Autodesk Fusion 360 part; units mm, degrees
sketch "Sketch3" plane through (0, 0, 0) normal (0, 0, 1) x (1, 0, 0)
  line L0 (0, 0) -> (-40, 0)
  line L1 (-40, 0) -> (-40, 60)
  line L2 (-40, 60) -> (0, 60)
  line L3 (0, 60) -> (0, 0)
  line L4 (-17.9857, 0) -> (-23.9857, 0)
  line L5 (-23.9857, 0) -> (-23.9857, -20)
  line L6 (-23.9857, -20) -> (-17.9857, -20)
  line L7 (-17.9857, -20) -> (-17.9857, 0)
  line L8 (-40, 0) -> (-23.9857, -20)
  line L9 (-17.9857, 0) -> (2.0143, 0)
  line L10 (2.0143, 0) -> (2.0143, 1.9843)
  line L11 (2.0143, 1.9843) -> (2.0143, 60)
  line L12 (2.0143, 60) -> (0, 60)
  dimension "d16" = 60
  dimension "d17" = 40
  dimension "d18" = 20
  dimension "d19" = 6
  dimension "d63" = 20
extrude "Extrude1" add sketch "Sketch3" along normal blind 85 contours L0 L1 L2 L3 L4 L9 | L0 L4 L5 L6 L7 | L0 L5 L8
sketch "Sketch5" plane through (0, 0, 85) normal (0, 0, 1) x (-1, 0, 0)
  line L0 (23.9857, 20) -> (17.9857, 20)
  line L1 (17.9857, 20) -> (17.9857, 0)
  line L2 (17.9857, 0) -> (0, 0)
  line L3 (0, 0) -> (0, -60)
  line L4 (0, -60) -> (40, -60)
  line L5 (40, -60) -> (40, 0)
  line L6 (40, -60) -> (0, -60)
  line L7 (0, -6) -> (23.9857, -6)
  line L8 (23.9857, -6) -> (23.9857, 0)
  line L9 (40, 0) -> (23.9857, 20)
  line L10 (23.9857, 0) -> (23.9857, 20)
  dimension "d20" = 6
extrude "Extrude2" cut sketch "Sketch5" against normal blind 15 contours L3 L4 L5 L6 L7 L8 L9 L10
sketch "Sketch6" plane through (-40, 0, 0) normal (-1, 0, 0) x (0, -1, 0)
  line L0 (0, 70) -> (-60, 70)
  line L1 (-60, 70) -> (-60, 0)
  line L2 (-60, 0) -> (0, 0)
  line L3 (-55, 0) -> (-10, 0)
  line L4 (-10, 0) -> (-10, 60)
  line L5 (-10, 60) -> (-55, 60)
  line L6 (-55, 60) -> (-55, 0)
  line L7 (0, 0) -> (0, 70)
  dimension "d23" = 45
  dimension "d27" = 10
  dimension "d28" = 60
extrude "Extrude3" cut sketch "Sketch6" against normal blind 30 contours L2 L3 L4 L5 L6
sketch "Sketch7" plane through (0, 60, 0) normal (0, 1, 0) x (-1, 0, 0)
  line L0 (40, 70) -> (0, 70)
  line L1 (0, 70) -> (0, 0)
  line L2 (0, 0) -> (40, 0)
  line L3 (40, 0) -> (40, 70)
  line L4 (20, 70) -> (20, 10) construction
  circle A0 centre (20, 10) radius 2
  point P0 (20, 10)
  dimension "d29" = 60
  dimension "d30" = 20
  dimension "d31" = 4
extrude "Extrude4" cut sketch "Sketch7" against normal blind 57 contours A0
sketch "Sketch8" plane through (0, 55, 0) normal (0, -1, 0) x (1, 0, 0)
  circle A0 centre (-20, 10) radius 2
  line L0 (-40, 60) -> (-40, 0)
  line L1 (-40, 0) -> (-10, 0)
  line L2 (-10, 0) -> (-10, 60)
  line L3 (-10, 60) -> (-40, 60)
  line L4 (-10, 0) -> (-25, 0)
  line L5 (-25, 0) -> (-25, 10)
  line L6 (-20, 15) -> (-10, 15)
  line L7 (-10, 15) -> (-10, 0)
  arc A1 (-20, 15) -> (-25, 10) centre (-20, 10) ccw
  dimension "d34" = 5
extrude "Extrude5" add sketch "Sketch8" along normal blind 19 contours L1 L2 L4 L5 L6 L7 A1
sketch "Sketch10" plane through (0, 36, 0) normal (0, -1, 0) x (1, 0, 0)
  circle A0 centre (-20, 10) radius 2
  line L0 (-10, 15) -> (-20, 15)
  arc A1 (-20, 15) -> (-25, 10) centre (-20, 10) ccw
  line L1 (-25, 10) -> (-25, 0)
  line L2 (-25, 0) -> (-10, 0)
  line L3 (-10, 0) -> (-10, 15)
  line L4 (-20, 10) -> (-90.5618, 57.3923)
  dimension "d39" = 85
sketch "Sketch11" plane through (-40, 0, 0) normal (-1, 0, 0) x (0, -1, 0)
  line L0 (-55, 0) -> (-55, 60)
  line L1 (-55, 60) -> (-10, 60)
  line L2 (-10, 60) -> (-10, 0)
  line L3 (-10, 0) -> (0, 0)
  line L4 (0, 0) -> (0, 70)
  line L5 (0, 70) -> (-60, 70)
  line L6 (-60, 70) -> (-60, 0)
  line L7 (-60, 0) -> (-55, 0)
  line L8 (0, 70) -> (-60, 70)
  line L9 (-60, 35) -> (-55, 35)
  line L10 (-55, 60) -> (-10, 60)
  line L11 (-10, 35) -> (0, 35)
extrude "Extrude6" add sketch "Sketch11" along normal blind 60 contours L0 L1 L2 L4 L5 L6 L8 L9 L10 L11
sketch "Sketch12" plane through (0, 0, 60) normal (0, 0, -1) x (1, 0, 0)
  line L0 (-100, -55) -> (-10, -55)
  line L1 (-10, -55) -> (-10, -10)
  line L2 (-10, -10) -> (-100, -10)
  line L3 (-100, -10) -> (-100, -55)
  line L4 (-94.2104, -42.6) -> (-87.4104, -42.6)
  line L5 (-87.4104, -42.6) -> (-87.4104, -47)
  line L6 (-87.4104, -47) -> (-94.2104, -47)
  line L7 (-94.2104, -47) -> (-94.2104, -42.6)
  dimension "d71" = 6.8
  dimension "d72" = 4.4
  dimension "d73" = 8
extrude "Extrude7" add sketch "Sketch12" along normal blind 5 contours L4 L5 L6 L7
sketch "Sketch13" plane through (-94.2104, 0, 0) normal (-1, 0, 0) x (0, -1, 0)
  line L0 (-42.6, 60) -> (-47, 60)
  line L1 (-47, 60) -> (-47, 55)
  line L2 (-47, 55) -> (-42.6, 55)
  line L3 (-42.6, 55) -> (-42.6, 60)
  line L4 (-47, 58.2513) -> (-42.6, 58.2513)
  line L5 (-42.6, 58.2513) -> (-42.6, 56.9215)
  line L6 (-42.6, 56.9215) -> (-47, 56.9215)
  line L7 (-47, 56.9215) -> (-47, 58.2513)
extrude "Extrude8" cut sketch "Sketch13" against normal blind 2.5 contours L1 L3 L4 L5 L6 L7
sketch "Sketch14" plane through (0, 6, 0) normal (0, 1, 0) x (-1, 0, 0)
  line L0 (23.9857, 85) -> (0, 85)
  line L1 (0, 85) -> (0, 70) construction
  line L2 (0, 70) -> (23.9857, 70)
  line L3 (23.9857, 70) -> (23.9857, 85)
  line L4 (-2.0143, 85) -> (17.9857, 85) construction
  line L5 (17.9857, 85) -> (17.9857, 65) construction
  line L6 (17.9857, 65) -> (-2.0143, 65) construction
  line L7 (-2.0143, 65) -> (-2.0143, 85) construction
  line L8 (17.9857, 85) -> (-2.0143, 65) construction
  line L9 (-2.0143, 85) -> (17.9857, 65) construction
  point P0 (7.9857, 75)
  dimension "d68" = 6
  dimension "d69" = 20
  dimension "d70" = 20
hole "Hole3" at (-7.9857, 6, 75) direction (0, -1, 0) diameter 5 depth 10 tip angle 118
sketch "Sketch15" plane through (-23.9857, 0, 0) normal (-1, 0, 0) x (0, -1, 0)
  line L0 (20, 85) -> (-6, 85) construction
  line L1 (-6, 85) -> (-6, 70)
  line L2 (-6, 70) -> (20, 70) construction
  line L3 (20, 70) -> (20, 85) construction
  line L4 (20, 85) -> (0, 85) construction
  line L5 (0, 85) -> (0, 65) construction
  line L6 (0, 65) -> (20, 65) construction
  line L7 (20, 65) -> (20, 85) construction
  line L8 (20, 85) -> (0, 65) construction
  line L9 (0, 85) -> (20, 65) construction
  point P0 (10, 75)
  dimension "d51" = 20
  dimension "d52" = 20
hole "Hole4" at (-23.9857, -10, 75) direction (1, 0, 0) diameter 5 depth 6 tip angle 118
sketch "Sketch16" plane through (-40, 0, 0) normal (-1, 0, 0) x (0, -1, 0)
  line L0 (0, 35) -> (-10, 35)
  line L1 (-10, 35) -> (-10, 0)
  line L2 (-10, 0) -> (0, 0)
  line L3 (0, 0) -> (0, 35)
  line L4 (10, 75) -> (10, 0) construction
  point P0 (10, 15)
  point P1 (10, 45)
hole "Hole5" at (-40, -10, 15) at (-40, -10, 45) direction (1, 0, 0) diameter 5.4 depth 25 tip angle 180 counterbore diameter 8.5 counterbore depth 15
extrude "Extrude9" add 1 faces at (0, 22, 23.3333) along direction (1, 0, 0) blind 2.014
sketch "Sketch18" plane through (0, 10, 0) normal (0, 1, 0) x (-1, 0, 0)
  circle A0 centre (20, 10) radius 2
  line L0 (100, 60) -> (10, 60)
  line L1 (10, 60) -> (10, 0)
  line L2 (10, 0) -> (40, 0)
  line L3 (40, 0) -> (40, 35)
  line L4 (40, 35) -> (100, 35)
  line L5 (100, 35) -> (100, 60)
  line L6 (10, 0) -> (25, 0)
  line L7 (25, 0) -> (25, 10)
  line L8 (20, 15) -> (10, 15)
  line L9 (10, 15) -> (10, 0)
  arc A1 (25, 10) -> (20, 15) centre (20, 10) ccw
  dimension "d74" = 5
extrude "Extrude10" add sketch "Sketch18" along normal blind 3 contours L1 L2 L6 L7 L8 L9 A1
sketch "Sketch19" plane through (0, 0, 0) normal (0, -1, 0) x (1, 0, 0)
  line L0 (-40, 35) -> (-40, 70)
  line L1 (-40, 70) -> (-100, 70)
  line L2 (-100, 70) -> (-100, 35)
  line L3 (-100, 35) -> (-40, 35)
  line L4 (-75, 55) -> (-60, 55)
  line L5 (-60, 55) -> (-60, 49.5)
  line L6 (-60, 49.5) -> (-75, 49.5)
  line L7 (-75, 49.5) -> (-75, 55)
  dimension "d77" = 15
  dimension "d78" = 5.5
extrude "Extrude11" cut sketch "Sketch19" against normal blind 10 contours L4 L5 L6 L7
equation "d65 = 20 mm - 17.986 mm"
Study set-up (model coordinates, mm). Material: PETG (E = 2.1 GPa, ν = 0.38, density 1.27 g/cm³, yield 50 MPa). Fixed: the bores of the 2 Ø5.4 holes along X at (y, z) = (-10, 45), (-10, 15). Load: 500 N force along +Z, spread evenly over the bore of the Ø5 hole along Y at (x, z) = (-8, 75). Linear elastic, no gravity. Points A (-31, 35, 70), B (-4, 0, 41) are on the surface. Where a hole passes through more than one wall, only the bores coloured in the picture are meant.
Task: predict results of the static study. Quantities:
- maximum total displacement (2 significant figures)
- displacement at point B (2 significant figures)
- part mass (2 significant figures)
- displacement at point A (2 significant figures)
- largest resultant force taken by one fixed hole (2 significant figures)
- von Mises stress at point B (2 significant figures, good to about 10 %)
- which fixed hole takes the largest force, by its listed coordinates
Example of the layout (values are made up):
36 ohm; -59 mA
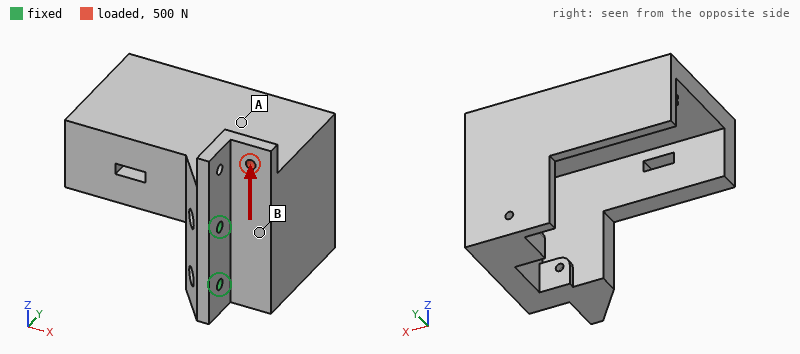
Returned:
0.22 mm; 0.076 mm; 230 g; 0.12 mm; 410 N; 1.3 MPa; (-10, 45)
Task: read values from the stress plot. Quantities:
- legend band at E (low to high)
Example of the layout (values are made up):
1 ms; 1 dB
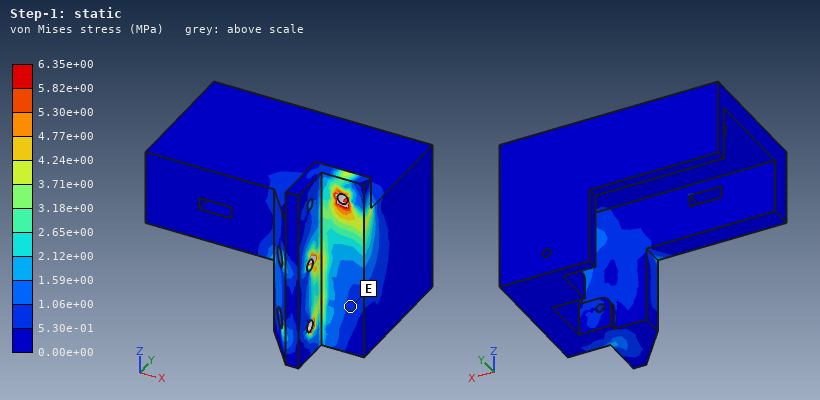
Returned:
5.30e-01 to 1.06e+00 MPa
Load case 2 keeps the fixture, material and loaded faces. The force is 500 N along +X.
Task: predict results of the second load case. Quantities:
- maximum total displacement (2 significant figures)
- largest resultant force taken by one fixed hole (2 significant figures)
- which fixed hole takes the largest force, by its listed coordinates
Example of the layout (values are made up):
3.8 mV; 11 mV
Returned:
1.2 mm; 900 N; (-10, 45)
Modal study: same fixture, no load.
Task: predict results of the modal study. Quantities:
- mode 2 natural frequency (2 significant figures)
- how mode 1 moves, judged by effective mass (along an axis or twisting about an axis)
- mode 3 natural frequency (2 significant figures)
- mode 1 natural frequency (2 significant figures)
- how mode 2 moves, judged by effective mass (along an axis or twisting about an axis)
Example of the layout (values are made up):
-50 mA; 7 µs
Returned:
380 Hz; along X; 630 Hz; 170 Hz; along Z
